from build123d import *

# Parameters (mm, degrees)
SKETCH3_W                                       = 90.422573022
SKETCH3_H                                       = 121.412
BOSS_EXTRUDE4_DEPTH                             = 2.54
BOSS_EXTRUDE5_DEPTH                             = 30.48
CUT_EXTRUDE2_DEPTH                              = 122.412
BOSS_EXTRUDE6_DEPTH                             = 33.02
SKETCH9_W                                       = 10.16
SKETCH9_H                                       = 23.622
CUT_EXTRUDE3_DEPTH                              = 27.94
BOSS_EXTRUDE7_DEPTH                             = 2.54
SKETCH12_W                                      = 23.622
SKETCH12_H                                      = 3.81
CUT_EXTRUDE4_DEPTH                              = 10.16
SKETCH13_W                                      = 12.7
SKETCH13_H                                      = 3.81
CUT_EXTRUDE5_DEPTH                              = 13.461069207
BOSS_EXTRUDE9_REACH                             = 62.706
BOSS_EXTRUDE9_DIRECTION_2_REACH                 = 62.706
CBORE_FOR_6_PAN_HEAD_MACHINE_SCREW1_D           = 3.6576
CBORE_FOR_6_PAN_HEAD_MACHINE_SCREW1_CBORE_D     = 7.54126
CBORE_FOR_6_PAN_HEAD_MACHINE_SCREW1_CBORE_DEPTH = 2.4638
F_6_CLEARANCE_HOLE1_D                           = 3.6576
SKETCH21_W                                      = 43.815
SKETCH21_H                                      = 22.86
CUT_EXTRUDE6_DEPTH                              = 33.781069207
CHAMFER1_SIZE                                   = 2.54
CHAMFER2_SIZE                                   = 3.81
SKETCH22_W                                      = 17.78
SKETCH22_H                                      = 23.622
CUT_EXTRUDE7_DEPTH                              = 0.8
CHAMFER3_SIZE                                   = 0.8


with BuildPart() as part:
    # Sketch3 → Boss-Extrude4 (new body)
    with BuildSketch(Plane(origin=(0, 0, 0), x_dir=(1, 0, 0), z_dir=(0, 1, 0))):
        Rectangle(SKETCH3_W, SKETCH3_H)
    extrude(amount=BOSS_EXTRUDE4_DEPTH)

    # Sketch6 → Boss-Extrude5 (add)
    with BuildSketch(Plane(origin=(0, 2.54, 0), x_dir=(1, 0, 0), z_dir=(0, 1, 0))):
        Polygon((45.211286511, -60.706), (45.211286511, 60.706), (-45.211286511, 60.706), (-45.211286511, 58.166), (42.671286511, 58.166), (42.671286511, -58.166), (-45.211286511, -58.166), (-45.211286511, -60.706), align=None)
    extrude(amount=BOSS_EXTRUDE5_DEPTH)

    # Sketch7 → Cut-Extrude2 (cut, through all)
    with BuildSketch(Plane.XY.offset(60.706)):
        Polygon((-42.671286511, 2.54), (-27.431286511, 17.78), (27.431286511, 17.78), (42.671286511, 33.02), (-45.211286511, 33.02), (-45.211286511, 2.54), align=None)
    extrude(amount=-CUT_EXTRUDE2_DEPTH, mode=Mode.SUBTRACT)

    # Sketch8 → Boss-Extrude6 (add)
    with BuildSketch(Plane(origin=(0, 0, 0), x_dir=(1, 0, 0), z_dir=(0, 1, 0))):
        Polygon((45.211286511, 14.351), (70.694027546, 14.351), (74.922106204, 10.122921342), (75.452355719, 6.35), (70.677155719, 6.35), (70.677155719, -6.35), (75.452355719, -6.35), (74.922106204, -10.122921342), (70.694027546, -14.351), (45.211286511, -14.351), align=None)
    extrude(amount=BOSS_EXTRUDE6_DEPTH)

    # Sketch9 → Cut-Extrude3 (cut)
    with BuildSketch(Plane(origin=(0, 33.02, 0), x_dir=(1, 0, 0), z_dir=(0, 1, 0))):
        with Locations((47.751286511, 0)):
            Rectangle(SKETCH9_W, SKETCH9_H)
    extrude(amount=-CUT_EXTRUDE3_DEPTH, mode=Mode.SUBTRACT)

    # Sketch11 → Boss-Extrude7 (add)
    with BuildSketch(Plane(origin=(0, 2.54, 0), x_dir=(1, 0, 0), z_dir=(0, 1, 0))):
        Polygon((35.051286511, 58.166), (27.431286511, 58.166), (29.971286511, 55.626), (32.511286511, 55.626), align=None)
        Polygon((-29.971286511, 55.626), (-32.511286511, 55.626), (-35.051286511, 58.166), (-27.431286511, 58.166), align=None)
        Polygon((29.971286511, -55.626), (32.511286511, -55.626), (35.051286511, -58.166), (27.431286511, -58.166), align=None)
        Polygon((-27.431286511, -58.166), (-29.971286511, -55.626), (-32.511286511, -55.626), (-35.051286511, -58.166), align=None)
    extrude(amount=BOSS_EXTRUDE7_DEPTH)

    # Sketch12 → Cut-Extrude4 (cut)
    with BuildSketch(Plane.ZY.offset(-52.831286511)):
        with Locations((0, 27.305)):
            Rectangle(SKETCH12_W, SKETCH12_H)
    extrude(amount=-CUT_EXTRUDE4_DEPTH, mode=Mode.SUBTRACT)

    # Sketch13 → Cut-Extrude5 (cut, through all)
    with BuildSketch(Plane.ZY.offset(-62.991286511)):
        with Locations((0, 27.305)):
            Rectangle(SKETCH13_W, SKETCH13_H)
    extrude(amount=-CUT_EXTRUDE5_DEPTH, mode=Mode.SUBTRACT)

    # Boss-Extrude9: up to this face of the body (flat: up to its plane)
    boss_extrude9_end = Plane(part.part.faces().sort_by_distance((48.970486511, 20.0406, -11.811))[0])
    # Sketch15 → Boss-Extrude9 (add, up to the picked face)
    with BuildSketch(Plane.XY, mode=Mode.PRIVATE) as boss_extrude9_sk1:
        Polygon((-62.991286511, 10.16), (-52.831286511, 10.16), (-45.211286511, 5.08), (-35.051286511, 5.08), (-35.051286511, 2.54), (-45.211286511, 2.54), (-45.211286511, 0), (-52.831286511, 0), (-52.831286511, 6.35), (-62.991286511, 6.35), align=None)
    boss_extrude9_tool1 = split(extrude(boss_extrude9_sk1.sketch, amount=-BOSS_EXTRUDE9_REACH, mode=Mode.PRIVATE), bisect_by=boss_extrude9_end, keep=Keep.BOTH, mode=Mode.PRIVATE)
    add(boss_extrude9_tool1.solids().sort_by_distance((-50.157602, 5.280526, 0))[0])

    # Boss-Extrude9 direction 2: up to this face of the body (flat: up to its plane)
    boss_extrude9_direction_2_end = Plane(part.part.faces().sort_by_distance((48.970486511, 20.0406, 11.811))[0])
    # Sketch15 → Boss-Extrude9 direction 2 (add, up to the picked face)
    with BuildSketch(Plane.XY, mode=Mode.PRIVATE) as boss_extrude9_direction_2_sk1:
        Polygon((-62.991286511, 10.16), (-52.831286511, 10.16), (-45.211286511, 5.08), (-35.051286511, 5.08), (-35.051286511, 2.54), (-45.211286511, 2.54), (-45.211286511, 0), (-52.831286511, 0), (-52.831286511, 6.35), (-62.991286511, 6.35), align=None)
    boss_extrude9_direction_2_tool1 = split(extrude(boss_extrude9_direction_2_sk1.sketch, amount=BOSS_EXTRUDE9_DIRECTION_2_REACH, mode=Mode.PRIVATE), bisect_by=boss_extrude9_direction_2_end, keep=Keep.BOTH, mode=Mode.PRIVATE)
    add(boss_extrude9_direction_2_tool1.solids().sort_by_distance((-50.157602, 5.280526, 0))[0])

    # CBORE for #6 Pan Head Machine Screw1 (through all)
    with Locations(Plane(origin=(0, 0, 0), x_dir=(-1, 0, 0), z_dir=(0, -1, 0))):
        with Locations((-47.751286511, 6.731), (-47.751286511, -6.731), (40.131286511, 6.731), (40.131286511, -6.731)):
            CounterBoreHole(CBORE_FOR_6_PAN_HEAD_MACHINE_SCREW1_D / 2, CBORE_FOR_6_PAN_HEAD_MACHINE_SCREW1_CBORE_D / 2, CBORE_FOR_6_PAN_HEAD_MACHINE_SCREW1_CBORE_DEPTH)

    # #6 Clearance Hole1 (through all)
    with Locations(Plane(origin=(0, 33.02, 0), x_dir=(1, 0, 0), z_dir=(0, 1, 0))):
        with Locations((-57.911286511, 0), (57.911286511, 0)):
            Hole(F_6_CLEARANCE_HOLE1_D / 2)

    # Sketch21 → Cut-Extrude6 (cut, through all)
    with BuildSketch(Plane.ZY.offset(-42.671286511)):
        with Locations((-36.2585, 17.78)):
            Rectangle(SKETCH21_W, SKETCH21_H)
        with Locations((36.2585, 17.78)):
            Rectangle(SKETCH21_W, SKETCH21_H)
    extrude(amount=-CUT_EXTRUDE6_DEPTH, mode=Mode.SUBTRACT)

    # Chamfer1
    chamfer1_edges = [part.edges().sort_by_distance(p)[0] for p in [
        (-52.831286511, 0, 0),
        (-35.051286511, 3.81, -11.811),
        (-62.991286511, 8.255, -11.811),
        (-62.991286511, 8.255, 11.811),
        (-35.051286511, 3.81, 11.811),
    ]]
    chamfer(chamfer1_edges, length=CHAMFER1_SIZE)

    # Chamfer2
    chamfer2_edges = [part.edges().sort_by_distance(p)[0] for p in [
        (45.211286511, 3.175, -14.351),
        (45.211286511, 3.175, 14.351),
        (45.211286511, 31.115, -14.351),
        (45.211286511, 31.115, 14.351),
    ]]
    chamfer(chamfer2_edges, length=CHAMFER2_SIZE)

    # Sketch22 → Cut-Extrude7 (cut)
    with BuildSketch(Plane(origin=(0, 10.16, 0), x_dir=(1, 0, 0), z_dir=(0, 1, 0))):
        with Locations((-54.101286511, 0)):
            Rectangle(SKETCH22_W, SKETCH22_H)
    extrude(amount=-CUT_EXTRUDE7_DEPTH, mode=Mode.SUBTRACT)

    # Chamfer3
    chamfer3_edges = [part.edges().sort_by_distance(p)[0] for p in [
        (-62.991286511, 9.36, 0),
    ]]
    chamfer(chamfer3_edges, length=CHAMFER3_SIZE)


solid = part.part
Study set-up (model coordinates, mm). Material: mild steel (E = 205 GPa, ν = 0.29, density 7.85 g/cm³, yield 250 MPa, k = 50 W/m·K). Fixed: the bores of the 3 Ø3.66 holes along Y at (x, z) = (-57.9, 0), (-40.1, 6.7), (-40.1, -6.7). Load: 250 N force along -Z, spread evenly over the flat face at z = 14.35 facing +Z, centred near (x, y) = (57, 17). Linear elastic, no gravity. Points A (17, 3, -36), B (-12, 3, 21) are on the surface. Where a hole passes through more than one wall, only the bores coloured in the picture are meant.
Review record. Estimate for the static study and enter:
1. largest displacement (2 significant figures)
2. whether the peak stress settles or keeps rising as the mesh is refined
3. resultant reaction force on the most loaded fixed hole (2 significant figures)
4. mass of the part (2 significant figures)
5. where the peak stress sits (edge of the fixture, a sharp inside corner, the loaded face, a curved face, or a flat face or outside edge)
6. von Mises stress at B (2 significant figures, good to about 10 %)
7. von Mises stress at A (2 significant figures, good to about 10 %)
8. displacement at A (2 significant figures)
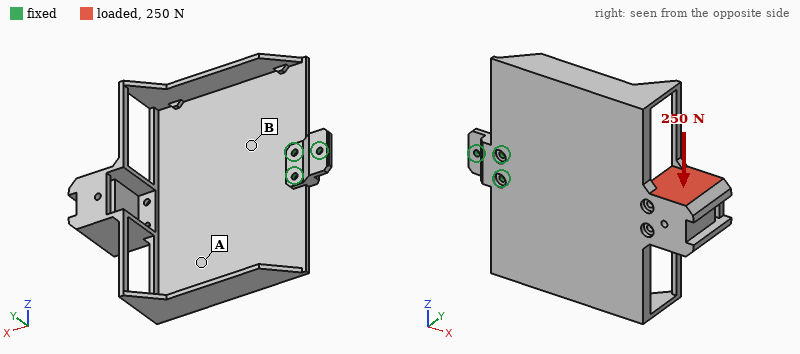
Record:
0.44 mm
keeps rising
980 N
460 g
edge of the fixture
26 MPa
13 MPa
0.18 mm
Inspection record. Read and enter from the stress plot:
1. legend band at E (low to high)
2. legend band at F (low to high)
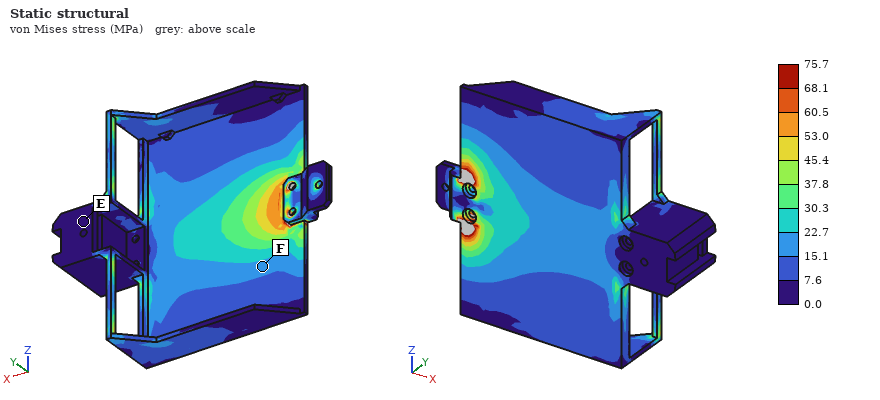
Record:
0.0 to 7.6 MPa
15.1 to 22.7 MPa
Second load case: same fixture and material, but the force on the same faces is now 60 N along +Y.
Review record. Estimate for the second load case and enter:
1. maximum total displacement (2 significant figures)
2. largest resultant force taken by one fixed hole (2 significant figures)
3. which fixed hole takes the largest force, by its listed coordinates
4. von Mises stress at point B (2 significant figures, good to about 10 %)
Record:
0.80 mm
300 N
(-57.9, 0)
23 MPa
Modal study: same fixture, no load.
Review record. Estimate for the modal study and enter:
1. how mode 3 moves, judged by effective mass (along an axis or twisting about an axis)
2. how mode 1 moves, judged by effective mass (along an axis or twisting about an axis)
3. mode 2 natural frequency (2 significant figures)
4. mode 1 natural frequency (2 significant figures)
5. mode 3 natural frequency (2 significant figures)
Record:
along Y
along Y
220 Hz
100 Hz
550 Hz
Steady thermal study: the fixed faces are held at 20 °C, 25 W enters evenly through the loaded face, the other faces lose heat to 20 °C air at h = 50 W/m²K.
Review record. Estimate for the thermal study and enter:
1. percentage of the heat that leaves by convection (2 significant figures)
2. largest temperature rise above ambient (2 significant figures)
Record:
97 %
61 K
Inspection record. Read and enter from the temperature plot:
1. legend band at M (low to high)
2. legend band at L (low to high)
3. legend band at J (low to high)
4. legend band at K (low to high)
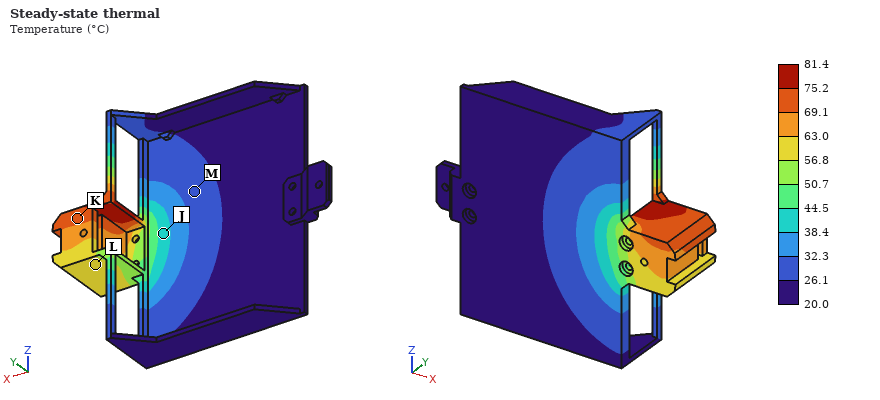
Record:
26.1 to 32.3 °C
56.8 to 63.0 °C
38.4 to 44.5 °C
69.1 to 75.2 °C
